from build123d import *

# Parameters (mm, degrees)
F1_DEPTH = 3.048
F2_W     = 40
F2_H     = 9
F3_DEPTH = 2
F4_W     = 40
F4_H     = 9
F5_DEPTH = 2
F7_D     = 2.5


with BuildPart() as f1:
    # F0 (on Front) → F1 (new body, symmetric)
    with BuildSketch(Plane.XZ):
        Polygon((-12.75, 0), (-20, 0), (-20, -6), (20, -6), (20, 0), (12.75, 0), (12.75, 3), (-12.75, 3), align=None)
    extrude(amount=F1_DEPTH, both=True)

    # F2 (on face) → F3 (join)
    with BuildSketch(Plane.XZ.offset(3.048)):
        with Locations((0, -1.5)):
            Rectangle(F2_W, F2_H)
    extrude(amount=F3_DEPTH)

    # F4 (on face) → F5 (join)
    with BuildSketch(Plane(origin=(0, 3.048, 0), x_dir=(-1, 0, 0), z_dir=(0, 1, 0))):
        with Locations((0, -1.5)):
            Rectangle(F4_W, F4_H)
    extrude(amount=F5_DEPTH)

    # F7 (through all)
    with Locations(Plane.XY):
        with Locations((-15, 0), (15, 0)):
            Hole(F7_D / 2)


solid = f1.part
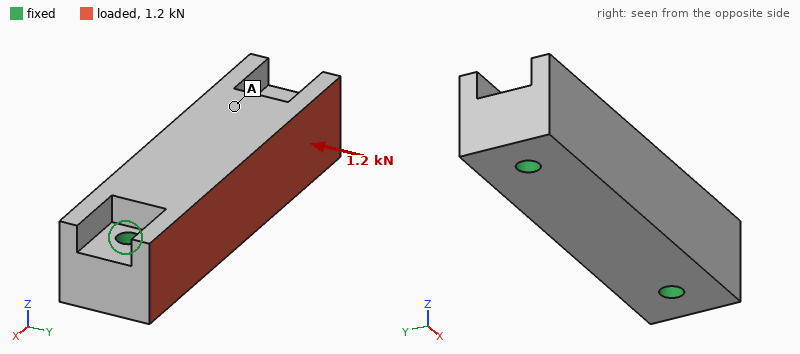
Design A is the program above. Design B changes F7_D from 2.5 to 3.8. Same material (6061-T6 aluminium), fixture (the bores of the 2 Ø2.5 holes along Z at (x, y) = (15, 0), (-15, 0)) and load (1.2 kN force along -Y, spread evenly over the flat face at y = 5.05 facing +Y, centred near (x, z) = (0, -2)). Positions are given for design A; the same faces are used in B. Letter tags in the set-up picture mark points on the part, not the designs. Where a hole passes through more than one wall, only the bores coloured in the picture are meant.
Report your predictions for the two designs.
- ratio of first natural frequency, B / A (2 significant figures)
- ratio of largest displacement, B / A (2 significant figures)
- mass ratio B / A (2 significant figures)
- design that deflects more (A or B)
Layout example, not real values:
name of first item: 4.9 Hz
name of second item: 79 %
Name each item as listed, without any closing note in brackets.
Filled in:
ratio of first natural frequency, B / A: 1.2
ratio of largest displacement, B / A: 0.73
mass ratio B / A: 0.98
design that deflects more: A
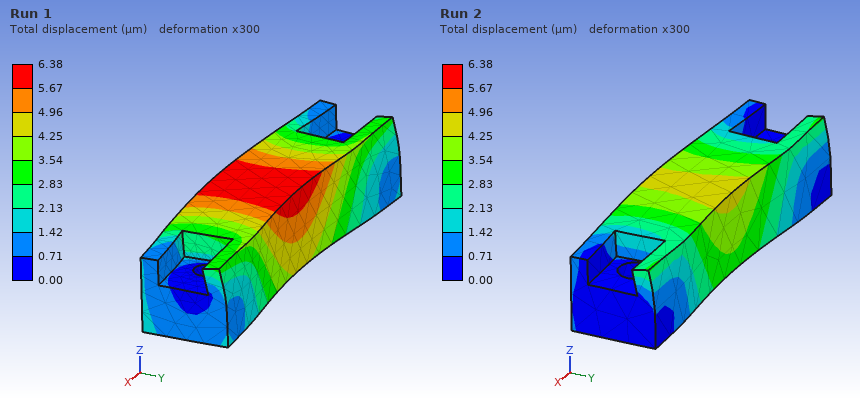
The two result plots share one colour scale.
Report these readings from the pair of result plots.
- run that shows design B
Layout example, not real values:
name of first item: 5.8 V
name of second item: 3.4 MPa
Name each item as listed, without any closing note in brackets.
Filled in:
run that shows design B: Run 2
